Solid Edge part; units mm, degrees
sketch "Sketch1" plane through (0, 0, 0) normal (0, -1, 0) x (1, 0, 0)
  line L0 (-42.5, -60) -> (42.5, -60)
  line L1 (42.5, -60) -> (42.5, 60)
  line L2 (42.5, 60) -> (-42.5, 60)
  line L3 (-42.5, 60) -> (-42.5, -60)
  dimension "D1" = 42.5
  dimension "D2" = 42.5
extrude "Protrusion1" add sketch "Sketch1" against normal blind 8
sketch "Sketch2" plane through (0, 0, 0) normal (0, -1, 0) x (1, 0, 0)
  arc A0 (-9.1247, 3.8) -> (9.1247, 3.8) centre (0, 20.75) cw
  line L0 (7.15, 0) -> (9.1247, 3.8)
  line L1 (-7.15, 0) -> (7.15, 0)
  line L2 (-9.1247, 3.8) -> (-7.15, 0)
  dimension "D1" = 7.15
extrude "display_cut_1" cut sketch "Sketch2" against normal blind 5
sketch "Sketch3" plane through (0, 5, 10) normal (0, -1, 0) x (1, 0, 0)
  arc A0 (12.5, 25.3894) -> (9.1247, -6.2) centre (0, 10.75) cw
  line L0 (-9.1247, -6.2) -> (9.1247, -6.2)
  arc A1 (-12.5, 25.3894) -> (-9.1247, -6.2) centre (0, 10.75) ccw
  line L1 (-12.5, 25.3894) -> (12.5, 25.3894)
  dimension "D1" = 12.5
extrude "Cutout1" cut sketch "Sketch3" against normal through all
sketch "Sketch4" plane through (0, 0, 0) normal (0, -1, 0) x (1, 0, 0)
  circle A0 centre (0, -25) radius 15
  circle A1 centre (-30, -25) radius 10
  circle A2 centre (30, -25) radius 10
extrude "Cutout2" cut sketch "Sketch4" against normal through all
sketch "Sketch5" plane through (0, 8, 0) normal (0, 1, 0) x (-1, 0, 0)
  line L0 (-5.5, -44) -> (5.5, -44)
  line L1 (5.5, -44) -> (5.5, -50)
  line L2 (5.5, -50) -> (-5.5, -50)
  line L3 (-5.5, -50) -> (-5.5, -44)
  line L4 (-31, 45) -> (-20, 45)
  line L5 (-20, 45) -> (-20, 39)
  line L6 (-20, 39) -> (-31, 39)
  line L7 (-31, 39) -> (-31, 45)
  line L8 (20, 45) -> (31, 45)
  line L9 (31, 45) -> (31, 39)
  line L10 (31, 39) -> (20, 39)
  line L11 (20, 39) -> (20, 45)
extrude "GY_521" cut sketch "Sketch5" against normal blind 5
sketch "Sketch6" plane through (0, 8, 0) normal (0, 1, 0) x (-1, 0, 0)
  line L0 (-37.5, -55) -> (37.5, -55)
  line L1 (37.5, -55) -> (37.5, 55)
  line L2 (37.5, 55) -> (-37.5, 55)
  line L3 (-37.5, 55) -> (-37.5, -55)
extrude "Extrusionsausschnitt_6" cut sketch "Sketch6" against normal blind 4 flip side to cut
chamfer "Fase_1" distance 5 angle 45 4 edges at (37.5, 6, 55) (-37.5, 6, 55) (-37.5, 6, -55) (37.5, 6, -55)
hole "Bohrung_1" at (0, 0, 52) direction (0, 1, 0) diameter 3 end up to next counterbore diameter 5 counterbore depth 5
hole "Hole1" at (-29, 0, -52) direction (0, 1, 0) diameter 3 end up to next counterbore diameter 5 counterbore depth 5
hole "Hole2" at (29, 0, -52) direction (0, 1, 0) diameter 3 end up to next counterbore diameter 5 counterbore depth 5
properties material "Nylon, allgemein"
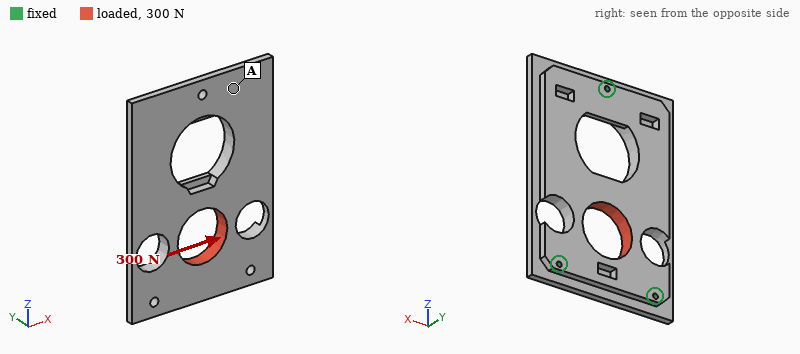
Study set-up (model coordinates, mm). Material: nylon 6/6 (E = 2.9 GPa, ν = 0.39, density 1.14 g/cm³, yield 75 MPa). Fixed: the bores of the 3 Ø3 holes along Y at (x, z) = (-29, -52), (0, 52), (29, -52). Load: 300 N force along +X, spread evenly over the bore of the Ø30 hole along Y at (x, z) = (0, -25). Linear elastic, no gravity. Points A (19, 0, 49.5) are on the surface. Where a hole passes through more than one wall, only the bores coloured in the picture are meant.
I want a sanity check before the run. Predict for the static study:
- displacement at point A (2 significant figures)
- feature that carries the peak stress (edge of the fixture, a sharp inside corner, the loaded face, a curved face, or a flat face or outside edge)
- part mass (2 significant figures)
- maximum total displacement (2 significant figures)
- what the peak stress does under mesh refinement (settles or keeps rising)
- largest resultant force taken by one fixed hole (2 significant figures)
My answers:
20 µm
edge of the fixture
60 g
63 µm
keeps rising
120 N
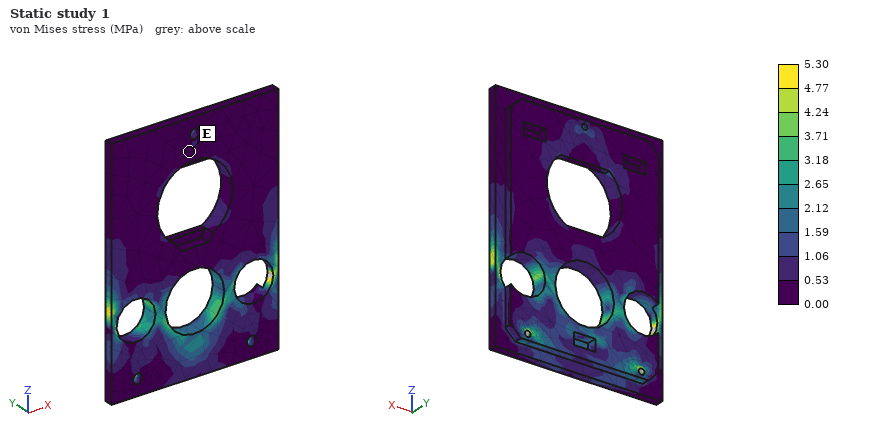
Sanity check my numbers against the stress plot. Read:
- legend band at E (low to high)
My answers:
0.00 to 0.53 MPa
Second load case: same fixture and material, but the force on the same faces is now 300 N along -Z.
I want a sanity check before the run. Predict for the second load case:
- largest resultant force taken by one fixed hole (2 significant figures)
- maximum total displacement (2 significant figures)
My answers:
120 N
55 µm
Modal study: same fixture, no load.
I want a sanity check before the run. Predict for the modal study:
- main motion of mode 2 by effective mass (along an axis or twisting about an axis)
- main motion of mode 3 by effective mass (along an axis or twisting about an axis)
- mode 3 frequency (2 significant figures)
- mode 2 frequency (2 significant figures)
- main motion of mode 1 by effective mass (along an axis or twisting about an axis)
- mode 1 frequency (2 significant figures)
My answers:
along Y
twisting about X
1200 Hz
570 Hz
twisting about Z
430 Hz
